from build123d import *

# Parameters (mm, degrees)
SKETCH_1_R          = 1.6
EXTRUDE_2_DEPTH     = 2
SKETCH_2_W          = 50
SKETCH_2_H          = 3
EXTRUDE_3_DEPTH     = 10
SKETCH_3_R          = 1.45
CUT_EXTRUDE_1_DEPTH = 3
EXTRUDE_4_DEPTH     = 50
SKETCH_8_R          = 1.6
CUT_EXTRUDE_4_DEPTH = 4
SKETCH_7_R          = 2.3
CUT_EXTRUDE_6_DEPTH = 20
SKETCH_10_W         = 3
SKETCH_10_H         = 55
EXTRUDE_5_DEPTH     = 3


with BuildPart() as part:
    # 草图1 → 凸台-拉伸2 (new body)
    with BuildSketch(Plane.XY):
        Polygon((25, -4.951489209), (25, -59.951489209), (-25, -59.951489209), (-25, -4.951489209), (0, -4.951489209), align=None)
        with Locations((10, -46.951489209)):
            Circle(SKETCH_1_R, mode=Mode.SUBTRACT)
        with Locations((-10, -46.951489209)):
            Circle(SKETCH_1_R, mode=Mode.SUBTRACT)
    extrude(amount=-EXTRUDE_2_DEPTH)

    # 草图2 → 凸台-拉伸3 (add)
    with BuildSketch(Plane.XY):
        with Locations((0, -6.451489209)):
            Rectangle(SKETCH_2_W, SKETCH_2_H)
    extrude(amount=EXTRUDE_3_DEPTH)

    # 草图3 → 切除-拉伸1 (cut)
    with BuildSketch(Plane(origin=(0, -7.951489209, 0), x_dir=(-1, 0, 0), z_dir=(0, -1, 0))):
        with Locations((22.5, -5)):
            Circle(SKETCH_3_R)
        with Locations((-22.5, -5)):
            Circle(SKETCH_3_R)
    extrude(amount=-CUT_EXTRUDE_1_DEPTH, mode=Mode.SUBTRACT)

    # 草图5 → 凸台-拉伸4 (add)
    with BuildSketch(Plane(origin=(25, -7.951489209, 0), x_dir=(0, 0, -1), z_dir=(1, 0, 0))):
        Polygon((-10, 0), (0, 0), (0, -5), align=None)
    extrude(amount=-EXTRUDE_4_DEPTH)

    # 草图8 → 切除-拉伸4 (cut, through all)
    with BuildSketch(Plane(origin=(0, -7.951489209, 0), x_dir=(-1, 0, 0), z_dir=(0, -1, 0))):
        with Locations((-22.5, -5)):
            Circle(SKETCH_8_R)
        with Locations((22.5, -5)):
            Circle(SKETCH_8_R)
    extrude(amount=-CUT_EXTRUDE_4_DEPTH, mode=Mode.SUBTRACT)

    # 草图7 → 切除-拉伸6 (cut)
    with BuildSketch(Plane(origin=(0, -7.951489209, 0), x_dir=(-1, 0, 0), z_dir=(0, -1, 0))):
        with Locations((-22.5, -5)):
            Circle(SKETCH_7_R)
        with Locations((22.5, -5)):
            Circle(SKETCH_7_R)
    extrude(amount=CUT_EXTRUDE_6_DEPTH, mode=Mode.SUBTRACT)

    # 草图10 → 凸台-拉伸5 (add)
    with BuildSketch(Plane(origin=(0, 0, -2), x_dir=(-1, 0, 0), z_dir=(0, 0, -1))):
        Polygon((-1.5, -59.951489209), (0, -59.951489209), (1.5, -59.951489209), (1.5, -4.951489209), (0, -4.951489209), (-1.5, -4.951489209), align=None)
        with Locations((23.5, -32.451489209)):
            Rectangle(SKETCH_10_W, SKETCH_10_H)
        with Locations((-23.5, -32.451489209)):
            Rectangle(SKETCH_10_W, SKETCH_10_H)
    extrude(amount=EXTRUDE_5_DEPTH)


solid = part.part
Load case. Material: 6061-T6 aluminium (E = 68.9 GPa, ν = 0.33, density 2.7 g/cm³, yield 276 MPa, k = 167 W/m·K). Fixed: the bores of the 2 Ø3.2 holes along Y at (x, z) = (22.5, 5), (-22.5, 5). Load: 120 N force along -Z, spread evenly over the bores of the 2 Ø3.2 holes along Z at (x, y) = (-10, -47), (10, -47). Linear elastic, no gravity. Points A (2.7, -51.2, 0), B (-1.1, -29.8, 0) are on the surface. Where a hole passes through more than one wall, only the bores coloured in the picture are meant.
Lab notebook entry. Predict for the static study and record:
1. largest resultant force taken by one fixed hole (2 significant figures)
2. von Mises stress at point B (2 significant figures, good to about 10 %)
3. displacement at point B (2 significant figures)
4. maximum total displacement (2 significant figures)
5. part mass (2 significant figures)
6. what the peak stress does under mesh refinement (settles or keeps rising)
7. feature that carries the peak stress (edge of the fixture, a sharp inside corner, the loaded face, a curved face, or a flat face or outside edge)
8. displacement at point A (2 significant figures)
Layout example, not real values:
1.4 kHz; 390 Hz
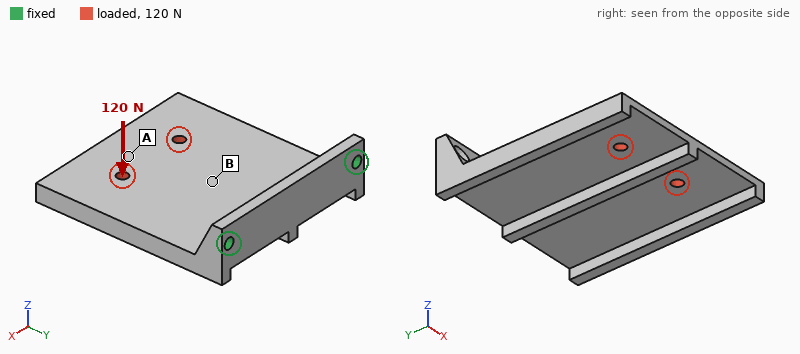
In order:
110 N; 18 MPa; 0.13 mm; 0.41 mm; 26 g; keeps rising; edge of the fixture; 0.33 mm
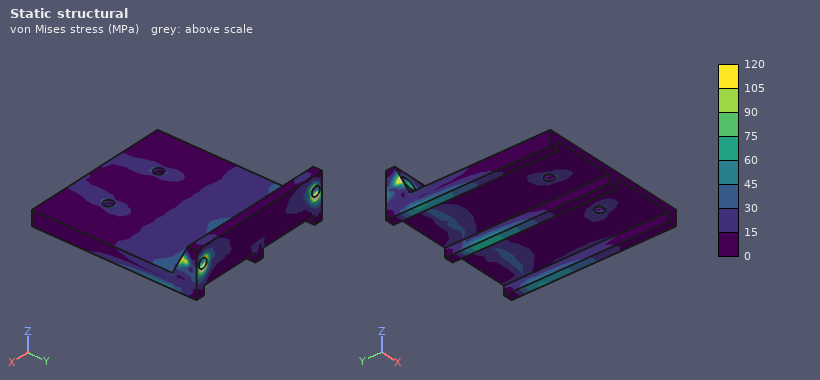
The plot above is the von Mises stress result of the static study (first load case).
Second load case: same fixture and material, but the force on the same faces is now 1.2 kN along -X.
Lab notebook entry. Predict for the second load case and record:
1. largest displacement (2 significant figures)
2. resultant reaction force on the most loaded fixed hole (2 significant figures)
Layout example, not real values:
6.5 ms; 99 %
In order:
0.10 mm; 1.3 kN
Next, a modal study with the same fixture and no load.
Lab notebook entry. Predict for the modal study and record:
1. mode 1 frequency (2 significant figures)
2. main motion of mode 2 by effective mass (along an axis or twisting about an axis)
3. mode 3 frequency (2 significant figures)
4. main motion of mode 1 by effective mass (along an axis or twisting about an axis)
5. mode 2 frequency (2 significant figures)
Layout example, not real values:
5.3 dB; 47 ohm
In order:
1100 Hz; twisting about Y; 4600 Hz; along Z; 2000 Hz
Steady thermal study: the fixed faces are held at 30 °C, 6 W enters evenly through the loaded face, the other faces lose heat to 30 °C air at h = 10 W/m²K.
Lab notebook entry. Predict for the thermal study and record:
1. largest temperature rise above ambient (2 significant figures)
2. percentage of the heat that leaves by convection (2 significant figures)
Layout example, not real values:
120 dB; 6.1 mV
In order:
14 K; 9.1 %
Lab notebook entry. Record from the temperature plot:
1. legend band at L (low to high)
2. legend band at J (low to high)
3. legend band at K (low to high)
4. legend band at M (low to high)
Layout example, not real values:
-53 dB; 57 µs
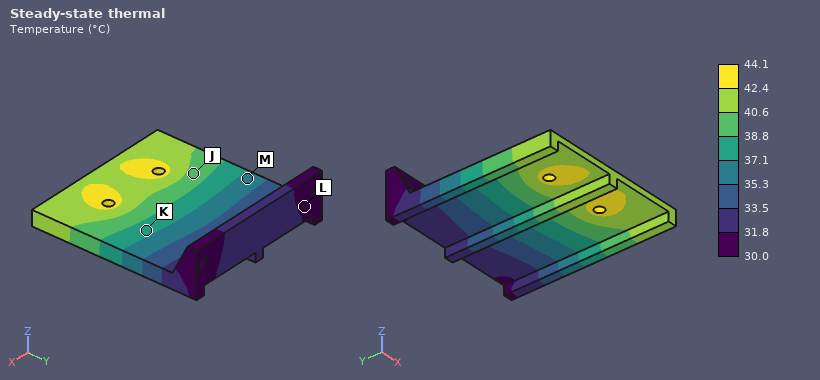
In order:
30.0 to 31.8 °C; 38.8 to 40.6 °C; 37.1 to 38.8 °C; 35.3 to 37.1 °C
